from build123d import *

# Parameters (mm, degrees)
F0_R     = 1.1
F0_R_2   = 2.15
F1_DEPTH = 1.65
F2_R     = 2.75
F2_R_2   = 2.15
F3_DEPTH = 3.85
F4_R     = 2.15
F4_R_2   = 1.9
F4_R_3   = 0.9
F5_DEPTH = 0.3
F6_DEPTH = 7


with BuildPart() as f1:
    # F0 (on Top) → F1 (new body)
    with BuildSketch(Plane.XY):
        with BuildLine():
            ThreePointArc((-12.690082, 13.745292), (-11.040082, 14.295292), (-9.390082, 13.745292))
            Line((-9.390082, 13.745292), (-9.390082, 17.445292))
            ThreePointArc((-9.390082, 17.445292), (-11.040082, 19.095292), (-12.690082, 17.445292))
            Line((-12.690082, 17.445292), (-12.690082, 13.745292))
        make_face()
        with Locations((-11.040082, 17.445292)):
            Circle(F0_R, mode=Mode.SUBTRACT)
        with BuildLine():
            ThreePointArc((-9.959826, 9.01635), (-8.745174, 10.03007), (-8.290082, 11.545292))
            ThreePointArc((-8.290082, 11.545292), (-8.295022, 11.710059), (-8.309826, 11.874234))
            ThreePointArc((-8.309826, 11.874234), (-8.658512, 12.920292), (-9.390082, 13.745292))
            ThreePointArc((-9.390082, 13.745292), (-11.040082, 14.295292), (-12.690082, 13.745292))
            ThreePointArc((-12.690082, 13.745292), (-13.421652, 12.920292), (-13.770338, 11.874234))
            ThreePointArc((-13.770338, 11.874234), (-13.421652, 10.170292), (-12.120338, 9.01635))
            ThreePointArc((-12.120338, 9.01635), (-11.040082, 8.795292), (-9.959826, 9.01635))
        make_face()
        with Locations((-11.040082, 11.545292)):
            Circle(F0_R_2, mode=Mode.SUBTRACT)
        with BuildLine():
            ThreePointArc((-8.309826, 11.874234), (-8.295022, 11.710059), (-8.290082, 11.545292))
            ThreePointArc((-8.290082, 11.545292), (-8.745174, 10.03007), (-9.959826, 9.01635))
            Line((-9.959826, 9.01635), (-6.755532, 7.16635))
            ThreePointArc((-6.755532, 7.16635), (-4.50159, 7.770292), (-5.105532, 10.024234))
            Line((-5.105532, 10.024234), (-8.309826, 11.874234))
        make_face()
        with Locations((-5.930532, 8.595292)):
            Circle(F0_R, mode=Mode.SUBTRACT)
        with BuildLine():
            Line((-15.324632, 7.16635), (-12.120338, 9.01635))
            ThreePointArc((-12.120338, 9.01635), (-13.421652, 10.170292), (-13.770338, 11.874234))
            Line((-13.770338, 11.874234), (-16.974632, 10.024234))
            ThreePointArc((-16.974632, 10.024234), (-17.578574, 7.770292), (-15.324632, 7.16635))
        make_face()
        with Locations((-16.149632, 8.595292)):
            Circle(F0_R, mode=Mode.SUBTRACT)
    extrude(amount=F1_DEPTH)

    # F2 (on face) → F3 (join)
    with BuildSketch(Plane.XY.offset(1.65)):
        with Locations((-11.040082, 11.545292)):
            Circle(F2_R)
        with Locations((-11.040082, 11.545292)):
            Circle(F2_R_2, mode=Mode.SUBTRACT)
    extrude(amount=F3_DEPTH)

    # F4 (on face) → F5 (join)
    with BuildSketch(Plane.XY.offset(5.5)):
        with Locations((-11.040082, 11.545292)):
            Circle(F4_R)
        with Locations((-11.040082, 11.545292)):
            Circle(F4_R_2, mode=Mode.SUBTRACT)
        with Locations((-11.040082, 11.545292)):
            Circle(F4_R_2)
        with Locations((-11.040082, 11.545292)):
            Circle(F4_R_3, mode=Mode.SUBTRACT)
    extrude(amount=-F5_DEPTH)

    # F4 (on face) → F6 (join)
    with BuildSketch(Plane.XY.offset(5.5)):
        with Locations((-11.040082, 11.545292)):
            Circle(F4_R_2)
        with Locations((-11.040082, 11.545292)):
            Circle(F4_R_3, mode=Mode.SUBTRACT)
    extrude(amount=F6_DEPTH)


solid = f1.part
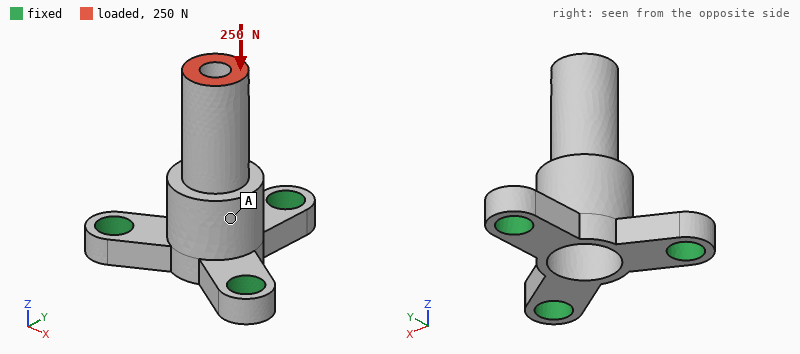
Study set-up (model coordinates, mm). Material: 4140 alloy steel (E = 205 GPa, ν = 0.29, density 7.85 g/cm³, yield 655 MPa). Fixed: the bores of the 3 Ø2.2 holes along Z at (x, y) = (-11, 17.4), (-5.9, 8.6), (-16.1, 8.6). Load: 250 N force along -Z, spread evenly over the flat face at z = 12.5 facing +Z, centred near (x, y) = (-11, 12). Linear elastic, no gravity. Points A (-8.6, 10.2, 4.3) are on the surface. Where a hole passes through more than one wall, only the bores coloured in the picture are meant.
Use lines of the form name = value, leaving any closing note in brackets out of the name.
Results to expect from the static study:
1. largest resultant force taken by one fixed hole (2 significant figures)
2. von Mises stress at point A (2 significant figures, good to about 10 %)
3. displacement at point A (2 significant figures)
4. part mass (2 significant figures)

largest resultant force taken by one fixed hole = 88 N
von Mises stress at point A = 23 MPa
displacement at point A = 2.3 µm
part mass = 1.4 g
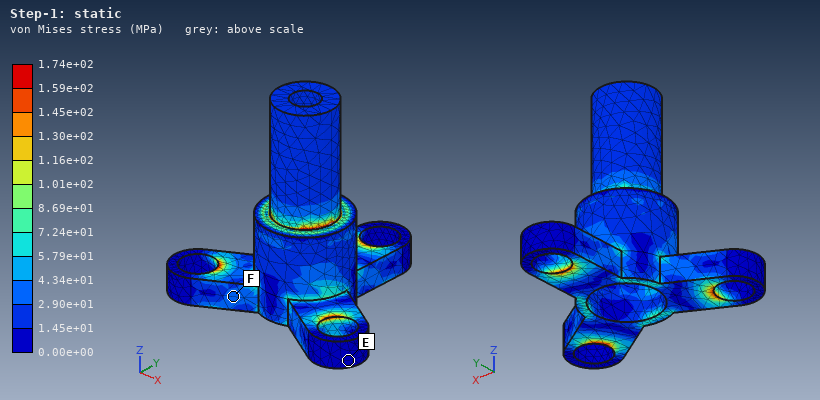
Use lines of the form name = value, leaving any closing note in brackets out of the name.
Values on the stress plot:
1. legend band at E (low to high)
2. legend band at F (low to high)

legend band at E = 0.00e+00 to 1.45e+01 MPa
legend band at F = 2.90e+01 to 4.34e+01 MPa
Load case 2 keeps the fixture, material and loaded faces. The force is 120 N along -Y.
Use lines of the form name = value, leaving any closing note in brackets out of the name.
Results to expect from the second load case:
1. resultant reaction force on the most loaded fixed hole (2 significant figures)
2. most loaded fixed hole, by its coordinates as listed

resultant reaction force on the most loaded fixed hole = 230 N
most loaded fixed hole, by its coordinates as listed = (-11, 17.4)
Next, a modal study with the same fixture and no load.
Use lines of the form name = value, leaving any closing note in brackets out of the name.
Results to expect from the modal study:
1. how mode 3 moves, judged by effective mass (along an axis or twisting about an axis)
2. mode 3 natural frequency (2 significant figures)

how mode 3 moves, judged by effective mass = along Z
mode 3 natural frequency = 49 kHz
